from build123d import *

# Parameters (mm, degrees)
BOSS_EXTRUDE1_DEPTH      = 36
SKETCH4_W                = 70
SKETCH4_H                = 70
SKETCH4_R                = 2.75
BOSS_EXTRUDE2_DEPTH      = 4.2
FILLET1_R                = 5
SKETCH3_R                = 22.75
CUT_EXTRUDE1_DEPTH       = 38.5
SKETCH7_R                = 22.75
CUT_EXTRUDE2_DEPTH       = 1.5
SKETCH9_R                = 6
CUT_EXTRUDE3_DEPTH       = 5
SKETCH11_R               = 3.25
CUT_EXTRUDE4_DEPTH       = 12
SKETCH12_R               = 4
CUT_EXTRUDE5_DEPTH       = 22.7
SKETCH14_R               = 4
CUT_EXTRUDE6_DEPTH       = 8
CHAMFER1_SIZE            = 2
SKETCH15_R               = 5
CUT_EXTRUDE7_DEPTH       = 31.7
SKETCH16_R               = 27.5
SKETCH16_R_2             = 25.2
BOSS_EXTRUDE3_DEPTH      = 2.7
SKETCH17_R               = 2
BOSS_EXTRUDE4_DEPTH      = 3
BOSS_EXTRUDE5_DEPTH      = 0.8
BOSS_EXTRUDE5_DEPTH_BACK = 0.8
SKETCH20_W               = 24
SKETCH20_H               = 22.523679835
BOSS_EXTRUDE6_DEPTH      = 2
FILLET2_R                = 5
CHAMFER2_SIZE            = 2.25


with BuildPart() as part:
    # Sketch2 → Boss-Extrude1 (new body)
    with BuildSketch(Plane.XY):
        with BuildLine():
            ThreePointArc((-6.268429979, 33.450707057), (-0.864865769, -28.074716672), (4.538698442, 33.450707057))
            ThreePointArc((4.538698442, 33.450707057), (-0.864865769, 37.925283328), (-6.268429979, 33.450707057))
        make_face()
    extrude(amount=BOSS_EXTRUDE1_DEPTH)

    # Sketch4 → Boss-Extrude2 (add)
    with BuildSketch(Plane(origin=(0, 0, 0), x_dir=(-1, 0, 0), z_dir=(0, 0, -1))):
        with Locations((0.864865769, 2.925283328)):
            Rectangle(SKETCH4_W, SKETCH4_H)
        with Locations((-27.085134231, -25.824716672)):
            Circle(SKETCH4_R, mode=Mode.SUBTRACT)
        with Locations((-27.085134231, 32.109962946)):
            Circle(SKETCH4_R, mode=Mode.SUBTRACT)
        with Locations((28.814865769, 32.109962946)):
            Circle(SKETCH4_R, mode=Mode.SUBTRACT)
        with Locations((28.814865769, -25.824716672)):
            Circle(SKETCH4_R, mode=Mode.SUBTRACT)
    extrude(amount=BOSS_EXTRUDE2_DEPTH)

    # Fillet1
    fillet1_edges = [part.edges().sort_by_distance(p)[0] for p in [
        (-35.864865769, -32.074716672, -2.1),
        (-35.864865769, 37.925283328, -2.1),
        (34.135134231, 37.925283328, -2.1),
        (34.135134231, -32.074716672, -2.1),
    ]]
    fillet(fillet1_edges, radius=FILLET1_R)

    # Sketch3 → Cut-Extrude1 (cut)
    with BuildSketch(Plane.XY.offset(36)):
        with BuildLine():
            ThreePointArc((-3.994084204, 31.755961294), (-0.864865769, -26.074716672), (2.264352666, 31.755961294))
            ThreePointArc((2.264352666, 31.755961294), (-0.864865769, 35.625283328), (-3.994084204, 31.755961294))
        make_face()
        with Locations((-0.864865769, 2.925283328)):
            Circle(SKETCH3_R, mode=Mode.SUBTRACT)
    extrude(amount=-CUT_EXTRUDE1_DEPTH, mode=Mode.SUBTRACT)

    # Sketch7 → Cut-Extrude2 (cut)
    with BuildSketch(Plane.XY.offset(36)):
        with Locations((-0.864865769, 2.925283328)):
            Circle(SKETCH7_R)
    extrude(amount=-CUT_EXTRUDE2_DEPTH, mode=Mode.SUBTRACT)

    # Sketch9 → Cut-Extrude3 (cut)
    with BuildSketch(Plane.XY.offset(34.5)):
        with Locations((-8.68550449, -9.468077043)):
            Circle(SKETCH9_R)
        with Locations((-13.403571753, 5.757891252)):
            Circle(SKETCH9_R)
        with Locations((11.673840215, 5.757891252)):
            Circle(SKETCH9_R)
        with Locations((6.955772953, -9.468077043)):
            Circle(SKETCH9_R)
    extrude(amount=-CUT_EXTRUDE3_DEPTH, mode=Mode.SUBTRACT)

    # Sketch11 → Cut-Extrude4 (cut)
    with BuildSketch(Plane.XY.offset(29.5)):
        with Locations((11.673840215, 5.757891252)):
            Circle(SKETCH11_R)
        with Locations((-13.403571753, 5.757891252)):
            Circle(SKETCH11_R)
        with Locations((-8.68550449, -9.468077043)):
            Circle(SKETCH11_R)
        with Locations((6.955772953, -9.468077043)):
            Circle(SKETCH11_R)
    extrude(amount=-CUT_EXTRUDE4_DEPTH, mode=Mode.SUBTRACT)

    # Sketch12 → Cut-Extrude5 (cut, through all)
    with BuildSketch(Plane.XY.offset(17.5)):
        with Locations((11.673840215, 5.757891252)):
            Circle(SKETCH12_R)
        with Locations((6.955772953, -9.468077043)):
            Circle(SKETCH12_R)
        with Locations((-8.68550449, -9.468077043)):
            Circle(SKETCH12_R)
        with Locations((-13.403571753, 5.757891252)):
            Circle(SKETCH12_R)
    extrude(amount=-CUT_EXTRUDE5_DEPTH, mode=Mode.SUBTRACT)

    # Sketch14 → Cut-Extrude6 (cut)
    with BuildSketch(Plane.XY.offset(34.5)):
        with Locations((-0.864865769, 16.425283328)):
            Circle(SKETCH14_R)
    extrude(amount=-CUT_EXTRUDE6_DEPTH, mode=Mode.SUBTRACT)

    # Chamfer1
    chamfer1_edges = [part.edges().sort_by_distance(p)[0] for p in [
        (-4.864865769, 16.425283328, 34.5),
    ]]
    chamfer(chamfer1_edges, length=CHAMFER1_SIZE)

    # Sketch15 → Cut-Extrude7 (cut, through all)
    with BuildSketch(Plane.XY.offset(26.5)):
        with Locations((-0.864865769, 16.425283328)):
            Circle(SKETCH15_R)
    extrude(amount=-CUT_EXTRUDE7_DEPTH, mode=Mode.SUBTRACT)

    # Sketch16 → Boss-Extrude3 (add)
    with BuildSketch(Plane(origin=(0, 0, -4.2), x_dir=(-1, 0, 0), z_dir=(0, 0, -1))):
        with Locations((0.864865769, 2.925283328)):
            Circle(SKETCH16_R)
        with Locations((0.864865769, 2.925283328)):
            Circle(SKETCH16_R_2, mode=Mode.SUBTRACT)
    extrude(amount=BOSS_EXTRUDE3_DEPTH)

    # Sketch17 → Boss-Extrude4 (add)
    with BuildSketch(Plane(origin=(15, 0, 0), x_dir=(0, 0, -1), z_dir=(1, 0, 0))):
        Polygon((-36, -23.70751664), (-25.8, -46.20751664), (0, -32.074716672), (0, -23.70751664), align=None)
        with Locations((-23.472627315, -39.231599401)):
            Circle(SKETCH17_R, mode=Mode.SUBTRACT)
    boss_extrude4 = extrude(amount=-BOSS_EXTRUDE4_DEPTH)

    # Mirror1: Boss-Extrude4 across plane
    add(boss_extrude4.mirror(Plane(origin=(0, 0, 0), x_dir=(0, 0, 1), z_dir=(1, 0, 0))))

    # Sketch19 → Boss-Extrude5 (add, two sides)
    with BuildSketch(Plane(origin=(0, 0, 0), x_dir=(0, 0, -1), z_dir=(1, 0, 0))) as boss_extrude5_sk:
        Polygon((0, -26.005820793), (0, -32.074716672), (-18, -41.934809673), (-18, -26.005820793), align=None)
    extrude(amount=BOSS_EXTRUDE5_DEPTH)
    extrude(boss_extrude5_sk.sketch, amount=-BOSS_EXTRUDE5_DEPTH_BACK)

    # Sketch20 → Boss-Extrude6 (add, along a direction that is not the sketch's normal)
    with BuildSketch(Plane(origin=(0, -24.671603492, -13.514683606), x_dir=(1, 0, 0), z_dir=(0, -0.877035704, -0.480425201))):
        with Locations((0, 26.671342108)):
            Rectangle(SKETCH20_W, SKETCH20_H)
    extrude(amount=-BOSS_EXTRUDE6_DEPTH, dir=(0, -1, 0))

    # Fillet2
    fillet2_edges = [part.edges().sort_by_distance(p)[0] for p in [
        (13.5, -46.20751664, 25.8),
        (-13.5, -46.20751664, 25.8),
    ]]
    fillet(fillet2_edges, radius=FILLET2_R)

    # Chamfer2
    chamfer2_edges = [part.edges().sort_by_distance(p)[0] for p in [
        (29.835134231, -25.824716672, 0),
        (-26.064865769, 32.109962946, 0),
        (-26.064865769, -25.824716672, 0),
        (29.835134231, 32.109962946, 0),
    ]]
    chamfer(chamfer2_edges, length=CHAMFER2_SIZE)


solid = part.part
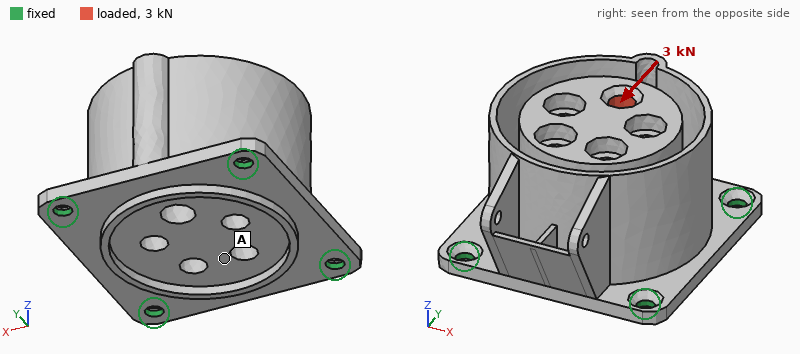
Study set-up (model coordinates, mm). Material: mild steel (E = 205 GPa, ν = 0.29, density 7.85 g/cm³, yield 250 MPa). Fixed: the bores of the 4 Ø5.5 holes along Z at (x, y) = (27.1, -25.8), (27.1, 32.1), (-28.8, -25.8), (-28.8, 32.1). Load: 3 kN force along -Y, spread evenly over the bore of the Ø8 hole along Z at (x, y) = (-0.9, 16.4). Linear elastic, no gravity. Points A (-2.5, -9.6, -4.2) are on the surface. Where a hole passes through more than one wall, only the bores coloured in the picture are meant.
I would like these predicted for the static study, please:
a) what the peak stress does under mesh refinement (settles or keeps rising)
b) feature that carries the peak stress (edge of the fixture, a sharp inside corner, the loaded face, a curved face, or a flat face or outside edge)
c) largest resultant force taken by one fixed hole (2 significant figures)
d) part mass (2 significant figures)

keeps rising
edge of the fixture
1.4 kN
640 g
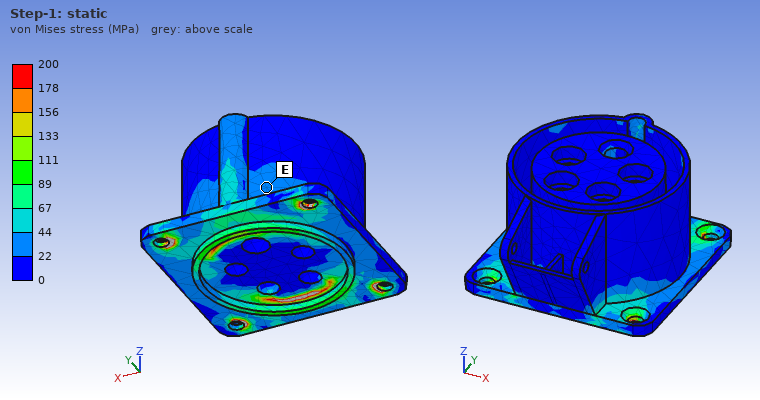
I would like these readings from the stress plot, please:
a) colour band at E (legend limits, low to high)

22 to 44 MPa
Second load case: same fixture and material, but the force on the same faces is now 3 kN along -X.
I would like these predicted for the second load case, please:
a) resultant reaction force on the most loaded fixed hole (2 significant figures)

1.5 kN
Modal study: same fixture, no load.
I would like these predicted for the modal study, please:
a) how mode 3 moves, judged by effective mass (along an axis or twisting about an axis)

along Z
